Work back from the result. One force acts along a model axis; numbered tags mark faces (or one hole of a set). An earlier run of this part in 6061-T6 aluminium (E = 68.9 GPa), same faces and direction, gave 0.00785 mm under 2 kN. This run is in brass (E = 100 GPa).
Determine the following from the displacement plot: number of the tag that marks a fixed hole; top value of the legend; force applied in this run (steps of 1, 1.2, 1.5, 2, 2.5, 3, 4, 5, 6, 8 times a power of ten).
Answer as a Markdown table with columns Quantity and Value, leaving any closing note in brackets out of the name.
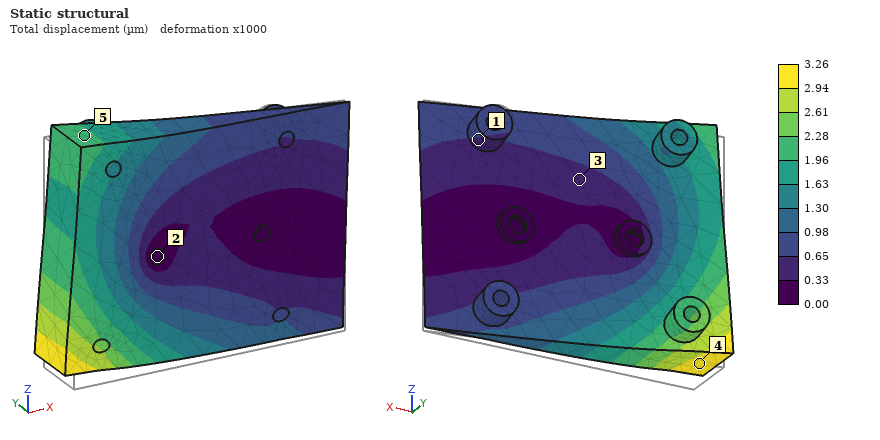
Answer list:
| Quantity | Value |
|---|---|
| number of the tag that marks a fixed hole | 2 |
| top value of the legend | 3.26 µm |
| force applied in this run | 1.2 kN |
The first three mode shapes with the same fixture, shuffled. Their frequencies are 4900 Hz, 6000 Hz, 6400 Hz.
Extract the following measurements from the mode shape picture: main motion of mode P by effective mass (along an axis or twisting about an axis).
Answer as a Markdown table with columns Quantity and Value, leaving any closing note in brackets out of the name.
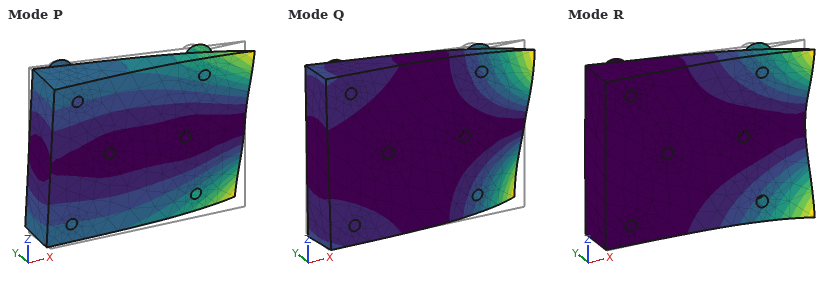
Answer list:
| Quantity | Value |
|---|---|
| main motion of mode P by effective mass | twisting about X |
